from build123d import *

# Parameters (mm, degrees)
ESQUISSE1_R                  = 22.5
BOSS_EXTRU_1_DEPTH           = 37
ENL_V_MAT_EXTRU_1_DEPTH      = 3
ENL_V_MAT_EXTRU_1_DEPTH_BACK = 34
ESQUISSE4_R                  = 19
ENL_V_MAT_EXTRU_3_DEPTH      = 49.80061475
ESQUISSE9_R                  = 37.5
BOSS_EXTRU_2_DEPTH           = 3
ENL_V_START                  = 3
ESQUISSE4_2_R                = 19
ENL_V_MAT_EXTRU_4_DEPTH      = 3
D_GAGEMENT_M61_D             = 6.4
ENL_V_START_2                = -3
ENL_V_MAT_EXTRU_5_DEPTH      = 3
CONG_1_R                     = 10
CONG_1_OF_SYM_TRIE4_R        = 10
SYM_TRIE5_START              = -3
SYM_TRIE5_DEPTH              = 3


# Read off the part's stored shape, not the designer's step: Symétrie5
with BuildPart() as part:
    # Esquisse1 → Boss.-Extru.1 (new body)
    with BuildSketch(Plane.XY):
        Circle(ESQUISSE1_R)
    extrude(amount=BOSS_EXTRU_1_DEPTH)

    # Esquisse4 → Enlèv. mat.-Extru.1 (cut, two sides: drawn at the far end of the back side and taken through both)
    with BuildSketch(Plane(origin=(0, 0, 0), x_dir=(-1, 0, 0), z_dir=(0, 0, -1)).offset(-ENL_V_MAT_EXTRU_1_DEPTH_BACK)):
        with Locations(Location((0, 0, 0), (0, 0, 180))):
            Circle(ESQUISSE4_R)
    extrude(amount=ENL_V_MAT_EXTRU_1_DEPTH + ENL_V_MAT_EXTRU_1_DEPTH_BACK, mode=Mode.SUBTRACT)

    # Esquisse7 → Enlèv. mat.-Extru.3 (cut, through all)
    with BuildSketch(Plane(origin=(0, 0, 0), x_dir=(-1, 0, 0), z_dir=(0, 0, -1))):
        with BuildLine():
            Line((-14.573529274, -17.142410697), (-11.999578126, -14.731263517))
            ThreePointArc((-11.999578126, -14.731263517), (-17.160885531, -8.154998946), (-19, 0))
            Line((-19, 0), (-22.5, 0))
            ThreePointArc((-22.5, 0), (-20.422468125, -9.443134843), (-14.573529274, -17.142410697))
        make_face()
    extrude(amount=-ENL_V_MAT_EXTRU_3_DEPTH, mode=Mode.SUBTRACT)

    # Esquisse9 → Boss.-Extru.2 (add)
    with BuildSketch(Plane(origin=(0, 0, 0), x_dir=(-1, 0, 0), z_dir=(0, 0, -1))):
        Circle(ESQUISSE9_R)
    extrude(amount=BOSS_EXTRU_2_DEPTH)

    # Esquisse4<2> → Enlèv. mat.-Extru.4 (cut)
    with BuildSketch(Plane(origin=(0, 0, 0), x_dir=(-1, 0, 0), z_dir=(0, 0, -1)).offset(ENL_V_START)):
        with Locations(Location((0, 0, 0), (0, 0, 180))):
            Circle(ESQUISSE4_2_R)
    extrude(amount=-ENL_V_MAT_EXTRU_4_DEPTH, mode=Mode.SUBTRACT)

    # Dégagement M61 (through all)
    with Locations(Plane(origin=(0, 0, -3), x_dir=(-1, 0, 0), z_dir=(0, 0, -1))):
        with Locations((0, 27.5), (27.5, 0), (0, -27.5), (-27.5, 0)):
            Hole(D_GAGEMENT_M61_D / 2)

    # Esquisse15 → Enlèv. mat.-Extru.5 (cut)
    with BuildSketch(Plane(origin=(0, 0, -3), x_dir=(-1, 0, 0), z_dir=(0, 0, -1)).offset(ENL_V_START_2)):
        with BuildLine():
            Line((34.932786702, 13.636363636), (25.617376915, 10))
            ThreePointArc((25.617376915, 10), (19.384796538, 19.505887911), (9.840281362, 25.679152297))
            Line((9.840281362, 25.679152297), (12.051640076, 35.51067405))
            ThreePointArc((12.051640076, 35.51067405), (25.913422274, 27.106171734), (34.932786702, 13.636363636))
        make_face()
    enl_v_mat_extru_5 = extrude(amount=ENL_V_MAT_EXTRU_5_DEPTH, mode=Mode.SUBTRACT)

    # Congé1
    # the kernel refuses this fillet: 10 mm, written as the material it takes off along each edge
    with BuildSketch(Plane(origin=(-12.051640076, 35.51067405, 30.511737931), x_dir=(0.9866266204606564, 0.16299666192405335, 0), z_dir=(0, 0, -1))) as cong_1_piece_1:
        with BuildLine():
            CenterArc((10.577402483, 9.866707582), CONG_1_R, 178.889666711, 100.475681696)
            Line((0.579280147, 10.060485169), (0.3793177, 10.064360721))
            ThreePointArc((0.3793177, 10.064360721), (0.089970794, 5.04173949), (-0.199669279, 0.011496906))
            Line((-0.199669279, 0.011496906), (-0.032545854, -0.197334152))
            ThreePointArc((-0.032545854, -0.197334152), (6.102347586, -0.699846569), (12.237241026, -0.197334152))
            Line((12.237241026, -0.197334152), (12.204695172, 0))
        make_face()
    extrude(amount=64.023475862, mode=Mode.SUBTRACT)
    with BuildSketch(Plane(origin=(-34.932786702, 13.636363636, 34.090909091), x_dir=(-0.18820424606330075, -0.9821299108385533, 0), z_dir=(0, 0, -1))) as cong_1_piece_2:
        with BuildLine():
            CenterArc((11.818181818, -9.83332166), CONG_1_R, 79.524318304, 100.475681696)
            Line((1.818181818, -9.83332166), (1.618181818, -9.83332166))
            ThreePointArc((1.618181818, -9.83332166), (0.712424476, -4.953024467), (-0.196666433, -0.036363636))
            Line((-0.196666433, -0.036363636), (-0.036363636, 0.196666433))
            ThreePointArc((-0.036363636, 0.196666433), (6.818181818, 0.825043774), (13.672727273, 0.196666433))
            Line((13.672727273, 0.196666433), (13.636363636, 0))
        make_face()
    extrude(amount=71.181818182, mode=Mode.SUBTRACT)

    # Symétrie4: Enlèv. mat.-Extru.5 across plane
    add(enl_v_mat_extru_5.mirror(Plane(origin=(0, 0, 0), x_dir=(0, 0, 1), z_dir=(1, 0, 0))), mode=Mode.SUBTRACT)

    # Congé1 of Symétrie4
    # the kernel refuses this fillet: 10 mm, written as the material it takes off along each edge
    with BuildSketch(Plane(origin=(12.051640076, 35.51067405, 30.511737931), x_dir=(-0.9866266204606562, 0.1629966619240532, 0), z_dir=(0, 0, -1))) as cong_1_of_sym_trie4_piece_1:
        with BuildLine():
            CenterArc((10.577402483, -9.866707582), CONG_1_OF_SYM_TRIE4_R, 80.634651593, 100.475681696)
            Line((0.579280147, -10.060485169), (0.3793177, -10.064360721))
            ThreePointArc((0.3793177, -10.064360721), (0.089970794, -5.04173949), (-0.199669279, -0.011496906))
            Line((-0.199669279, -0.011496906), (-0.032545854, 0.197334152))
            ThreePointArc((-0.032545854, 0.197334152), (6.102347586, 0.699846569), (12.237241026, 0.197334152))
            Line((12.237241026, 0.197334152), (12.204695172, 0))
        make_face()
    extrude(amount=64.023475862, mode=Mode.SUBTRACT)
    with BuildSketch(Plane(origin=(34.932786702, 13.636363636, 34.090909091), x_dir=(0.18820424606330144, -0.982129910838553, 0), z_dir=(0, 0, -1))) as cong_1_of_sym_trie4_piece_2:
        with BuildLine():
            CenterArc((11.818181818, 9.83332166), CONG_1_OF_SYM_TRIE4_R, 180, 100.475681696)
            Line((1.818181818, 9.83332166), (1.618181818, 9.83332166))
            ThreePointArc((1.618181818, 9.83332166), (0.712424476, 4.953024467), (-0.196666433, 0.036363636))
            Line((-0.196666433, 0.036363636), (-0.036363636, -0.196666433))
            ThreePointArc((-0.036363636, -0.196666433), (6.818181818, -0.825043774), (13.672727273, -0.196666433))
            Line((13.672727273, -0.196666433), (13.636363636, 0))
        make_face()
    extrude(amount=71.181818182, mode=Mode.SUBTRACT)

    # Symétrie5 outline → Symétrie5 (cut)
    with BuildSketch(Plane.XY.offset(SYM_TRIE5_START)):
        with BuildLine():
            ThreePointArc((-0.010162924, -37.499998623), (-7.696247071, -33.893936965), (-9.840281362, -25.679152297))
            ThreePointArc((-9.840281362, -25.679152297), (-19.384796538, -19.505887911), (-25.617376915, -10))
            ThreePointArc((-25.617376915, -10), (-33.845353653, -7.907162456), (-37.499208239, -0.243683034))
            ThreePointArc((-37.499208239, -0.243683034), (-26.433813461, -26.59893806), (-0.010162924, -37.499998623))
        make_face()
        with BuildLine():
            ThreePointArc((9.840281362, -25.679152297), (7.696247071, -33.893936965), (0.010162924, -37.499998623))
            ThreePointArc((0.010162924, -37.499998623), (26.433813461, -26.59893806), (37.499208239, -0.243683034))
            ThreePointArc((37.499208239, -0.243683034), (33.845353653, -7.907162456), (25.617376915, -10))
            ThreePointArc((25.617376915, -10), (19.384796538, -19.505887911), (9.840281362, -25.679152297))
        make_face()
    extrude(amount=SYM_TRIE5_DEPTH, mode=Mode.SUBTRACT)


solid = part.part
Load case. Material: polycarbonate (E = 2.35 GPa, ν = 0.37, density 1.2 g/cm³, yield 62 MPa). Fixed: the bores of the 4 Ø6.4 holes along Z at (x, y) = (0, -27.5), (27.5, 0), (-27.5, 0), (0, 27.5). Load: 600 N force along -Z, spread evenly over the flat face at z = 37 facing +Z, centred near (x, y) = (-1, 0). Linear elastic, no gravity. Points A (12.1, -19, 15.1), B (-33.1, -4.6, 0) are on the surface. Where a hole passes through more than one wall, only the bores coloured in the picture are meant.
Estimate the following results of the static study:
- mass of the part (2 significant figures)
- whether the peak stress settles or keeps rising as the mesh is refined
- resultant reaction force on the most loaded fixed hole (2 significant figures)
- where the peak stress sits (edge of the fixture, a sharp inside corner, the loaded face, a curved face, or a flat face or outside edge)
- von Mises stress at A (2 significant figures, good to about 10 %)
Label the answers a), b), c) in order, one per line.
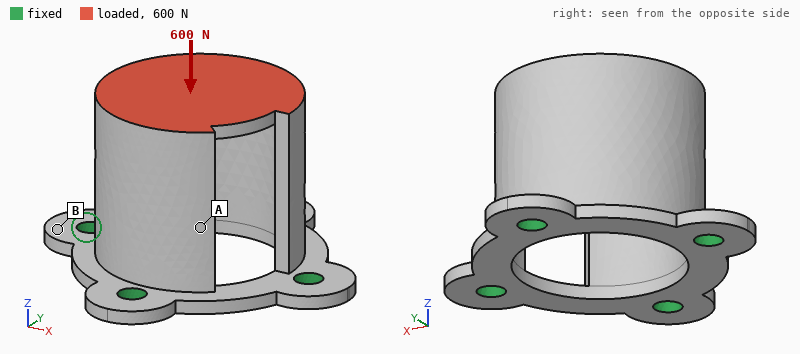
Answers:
a) 28 g
b) keeps rising
c) 190 N
d) edge of the fixture
e) 3.0 MPa
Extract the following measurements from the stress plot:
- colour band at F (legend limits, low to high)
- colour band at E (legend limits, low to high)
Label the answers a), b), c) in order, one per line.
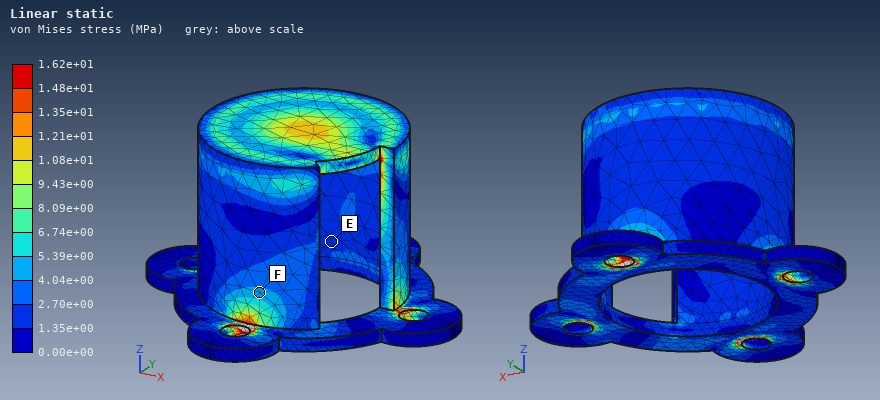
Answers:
a) 4.04e+00 to 5.39e+00 MPa
b) 1.35e+00 to 2.70e+00 MPa
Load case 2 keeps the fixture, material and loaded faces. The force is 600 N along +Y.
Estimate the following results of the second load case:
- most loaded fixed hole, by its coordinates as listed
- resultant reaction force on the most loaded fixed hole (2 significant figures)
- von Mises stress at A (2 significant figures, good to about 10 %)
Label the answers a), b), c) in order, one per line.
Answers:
a) (0, 27.5)
b) 760 N
c) 5.8 MPa
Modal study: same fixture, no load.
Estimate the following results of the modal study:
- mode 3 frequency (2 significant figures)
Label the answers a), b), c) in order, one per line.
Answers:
a) 2700 Hz
